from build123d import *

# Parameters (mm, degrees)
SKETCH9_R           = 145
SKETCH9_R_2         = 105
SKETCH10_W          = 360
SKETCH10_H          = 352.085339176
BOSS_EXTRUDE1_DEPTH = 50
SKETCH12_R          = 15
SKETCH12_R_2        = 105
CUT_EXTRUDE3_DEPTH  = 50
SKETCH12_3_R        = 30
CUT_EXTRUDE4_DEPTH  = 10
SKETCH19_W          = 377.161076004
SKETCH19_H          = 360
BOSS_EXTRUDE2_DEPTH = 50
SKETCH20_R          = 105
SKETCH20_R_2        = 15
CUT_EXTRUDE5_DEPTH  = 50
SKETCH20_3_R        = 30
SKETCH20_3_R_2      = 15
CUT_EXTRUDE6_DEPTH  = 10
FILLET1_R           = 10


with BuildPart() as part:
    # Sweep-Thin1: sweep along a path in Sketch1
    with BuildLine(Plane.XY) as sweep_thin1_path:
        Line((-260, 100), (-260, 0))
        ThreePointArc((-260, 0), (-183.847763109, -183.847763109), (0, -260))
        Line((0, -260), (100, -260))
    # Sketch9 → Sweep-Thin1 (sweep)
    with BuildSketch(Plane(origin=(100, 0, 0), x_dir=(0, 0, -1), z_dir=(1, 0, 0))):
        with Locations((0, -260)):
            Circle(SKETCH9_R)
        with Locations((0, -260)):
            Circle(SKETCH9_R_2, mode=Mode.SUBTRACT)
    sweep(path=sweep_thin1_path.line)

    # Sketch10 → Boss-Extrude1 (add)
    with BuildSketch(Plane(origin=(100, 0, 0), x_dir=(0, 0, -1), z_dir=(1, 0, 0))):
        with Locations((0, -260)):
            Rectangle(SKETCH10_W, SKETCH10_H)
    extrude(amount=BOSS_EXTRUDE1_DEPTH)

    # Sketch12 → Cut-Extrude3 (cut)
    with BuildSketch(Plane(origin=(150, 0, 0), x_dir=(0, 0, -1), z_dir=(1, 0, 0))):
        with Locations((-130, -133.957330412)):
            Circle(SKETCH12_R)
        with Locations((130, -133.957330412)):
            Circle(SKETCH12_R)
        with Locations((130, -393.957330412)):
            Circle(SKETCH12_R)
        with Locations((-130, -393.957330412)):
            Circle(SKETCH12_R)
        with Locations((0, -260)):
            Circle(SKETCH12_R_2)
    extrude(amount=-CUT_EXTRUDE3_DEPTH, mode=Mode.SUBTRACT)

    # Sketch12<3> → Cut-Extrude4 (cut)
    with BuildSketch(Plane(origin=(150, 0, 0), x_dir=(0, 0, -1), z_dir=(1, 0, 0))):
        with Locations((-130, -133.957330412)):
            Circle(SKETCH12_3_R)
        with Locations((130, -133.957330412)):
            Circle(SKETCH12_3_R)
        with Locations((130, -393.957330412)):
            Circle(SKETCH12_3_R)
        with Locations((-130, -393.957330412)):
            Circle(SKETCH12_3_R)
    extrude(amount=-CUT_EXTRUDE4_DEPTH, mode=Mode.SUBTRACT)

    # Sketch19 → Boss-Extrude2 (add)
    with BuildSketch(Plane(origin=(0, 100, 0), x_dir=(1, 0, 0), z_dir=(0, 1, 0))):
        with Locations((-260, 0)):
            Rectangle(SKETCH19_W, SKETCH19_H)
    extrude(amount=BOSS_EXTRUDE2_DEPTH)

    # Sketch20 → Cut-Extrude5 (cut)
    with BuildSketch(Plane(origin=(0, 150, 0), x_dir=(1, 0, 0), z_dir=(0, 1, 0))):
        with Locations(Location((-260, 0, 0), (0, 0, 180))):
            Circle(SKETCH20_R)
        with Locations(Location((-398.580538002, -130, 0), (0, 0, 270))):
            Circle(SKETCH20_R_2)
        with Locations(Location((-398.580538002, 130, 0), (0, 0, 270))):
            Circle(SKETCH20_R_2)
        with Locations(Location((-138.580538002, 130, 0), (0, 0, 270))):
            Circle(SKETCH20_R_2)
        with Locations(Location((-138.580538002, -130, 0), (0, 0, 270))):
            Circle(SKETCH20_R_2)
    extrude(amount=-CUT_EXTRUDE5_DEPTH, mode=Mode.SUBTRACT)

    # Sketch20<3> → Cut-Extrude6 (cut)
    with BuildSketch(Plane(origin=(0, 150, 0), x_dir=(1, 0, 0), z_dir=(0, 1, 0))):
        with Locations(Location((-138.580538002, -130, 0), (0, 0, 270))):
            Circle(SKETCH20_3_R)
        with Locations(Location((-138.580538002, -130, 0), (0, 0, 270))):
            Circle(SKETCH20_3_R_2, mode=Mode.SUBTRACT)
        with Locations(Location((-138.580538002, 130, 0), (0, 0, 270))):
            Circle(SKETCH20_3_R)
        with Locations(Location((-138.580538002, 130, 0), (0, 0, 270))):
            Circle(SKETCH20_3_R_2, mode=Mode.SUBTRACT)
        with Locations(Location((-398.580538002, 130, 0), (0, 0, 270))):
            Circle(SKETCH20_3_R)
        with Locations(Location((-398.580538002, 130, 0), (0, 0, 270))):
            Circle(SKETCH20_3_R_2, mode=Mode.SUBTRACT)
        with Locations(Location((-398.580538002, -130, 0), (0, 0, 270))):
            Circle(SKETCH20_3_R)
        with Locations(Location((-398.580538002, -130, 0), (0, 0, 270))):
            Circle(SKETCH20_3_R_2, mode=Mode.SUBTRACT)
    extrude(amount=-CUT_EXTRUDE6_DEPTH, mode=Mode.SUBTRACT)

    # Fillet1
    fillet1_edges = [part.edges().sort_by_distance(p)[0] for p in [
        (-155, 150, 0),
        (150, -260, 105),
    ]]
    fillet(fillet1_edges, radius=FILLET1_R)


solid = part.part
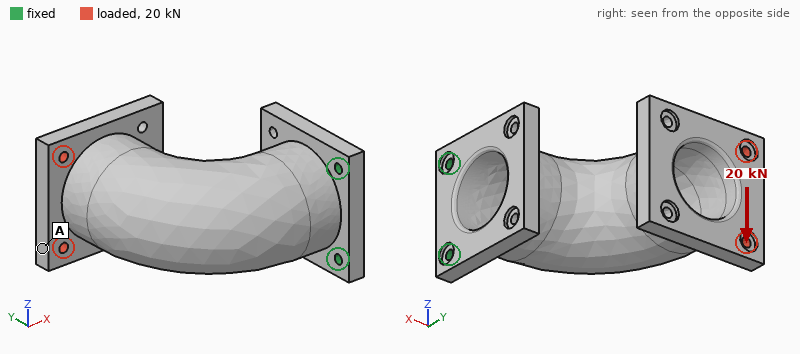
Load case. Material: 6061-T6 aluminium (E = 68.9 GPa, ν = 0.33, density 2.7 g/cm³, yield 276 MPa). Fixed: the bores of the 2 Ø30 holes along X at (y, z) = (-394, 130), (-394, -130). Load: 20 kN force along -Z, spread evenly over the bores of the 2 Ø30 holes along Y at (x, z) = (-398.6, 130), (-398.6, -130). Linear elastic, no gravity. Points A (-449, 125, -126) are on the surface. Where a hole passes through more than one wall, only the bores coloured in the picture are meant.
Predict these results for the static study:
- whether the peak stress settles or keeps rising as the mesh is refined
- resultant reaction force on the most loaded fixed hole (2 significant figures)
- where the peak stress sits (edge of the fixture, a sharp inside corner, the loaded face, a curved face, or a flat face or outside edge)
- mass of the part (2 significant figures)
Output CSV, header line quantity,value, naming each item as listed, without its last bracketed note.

quantity,value
whether the peak stress settles or keeps rising as the mesh is refined,keeps rising
resultant reaction force on the most loaded fixed hole,57 kN
where the peak stress sits,edge of the fixture
mass of the part,76 kg
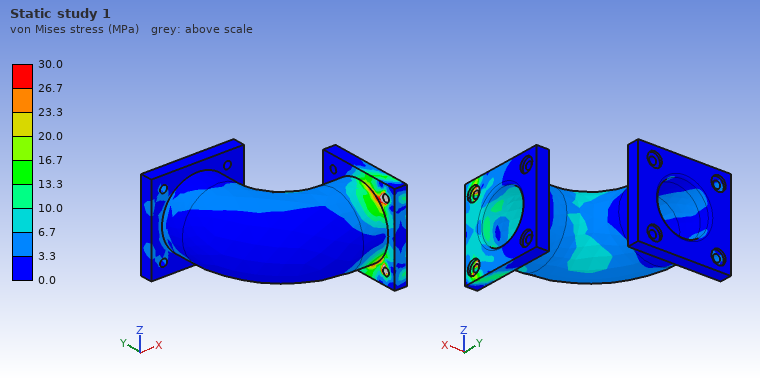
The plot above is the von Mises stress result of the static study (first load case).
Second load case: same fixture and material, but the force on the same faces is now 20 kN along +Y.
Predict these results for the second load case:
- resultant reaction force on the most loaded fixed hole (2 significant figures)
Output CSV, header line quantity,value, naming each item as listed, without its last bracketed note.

quantity,value
resultant reaction force on the most loaded fixed hole,11 kN
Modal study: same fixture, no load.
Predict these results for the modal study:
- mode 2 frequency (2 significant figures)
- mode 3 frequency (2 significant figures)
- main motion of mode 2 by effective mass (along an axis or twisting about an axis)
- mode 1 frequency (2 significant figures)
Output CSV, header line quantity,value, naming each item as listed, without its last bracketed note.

quantity,value
mode 2 frequency,210 Hz
mode 3 frequency,520 Hz
main motion of mode 2 by effective mass,along Z
mode 1 frequency,65 Hz
